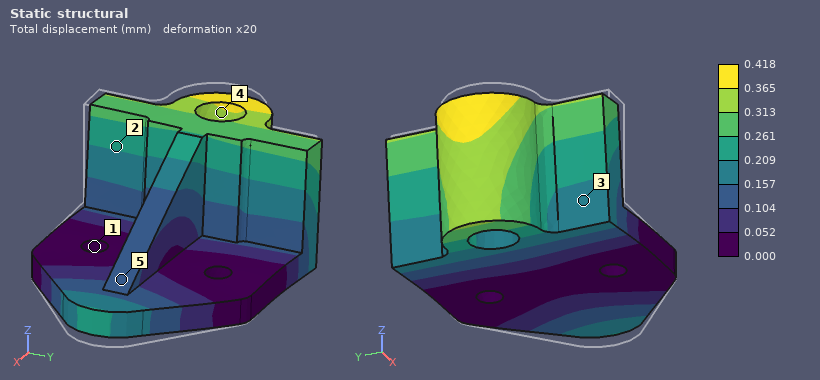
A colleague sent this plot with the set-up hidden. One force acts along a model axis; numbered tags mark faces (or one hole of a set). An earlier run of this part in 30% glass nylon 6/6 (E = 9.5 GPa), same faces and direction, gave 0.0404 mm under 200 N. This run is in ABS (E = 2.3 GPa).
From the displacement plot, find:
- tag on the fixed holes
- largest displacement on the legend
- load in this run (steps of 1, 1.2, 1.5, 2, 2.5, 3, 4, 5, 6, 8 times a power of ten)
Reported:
1
0.418 mm
500 N
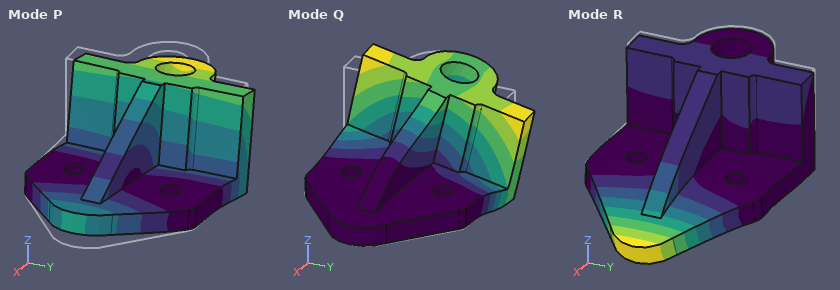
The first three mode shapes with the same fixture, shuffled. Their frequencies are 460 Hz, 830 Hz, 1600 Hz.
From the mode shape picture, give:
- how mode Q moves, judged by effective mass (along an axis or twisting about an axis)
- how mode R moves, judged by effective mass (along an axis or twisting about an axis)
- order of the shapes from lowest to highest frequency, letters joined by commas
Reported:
along Y
along Z
P, Q, R
